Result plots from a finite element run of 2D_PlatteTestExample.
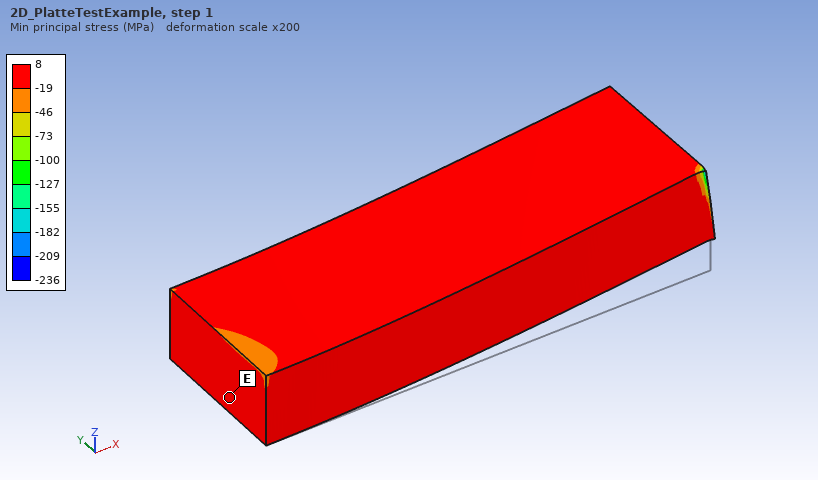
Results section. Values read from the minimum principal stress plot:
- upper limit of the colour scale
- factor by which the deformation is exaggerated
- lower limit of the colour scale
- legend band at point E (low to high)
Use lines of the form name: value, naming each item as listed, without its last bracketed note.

upper limit of the colour scale: 8 MPa
factor by which the deformation is exaggerated: 200
lower limit of the colour scale: -236 MPa
legend band at point E: -19 to 8 MPa
